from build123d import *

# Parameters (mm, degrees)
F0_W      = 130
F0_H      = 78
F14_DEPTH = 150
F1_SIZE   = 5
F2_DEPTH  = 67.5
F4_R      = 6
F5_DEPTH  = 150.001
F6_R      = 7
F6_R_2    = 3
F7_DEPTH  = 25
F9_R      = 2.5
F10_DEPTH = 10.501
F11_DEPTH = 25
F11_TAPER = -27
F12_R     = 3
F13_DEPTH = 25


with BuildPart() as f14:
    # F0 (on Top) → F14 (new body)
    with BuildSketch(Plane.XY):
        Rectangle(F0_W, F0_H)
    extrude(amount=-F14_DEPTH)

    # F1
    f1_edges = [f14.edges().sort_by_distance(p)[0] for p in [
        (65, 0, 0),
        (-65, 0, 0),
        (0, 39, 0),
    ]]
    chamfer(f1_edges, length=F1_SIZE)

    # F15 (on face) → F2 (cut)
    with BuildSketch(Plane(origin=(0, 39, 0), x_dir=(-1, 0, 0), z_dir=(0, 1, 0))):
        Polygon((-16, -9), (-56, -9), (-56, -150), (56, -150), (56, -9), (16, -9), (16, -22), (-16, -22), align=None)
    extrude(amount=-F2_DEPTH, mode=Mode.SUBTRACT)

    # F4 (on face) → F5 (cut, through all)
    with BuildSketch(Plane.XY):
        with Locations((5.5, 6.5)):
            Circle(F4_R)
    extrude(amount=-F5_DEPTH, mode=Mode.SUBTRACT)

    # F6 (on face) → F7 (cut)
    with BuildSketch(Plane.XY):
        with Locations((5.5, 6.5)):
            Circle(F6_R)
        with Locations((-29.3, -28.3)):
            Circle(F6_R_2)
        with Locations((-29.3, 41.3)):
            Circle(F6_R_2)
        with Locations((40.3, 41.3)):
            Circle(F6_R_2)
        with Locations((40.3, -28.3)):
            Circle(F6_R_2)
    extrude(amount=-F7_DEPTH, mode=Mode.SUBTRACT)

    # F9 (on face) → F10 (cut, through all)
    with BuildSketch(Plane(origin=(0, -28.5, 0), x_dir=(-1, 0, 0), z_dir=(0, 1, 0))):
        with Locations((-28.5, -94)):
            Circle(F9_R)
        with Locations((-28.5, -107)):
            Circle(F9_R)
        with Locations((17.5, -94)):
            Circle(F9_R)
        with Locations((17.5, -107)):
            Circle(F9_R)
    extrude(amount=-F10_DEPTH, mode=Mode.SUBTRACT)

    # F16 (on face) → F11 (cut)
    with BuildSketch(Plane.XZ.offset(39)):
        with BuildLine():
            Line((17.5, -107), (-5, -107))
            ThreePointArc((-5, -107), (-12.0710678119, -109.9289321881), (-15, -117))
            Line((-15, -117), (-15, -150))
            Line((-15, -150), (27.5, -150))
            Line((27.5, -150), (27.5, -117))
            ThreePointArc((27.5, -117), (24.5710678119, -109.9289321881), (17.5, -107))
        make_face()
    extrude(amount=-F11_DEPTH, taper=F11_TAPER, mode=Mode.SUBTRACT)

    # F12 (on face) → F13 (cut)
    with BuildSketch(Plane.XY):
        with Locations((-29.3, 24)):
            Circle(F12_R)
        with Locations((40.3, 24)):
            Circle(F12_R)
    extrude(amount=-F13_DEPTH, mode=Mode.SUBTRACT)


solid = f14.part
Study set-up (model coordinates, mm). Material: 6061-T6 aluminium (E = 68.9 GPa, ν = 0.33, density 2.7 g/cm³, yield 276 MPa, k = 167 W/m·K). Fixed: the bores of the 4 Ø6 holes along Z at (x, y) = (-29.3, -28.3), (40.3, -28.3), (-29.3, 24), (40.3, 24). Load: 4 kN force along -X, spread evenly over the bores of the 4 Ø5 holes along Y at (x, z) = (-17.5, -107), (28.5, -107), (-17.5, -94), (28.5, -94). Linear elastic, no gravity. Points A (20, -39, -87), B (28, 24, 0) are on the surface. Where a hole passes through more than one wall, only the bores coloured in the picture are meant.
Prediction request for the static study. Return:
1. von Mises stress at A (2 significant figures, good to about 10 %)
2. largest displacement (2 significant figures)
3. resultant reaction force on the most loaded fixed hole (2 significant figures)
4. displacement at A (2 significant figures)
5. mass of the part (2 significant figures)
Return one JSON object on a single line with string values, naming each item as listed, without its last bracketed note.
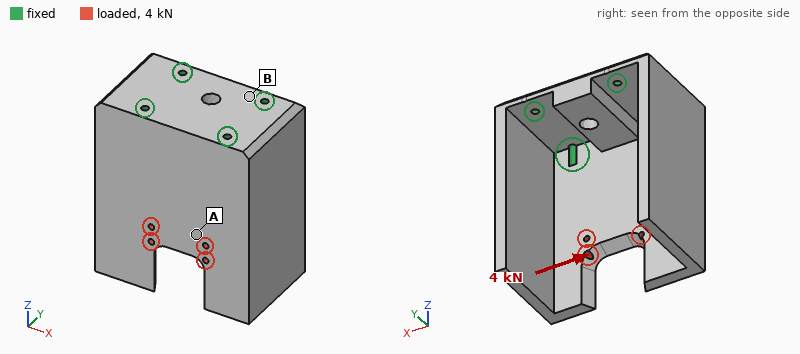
{"von Mises stress at A": "6.3 MPa", "largest displacement": "50 µm", "resultant reaction force on the most loaded fixed hole": "4.4 kN", "displacement at A": "20 µm", "mass of the part": "1.2 kg"}
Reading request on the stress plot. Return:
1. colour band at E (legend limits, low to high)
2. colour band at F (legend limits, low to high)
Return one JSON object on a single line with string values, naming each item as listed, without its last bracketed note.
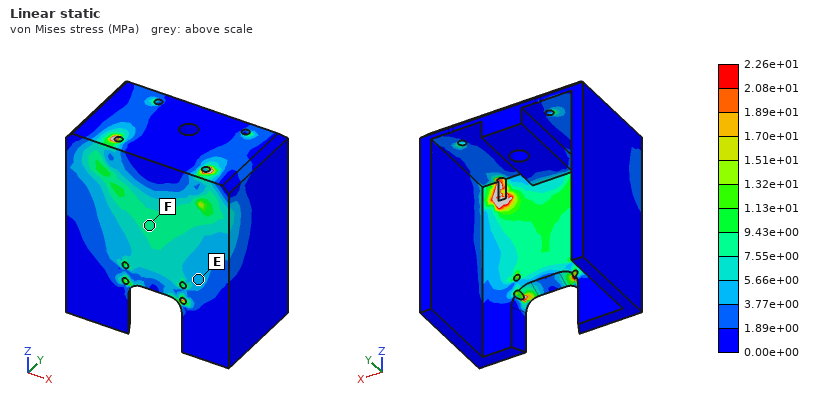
{"colour band at E": "3.77e+00 to 5.66e+00 MPa", "colour band at F": "7.55e+00 to 9.43e+00 MPa"}
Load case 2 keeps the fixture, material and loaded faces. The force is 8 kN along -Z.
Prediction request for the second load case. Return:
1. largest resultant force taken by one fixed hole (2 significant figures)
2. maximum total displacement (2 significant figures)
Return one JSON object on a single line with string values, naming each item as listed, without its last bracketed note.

{"largest resultant force taken by one fixed hole": "4.2 kN", "maximum total displacement": "27 µm"}
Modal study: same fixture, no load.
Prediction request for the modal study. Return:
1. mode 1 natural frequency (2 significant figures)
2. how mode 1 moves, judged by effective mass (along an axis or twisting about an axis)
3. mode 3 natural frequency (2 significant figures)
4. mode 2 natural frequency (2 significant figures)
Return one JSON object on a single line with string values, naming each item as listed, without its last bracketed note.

{"mode 1 natural frequency": "950 Hz", "how mode 1 moves, judged by effective mass": "along Y", "mode 3 natural frequency": "1200 Hz", "mode 2 natural frequency": "1100 Hz"}
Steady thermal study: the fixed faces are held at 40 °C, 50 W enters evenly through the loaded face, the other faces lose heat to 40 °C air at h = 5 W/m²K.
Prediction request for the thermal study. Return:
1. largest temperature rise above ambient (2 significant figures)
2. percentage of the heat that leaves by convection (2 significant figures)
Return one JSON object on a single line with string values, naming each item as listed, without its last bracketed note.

{"largest temperature rise above ambient": "18 K", "percentage of the heat that leaves by convection": "6.0 %"}
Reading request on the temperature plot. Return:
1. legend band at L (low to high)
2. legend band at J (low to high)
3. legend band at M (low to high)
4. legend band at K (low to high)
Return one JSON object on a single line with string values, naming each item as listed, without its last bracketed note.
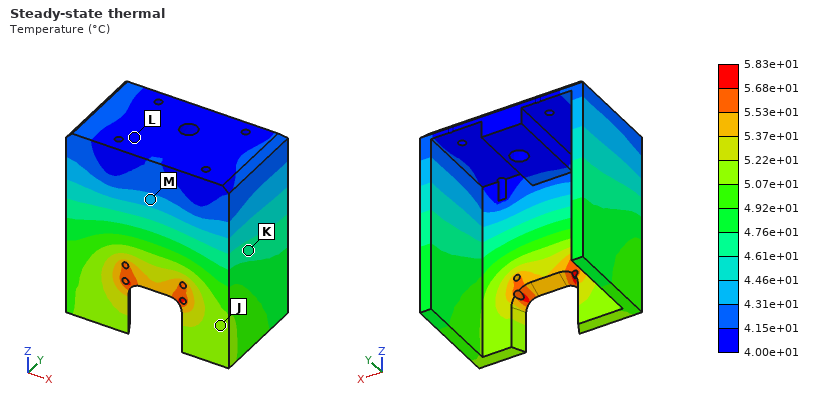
{"legend band at L": "4.00e+01 to 4.15e+01 °C", "legend band at J": "5.07e+01 to 5.22e+01 °C", "legend band at M": "4.31e+01 to 4.46e+01 °C", "legend band at K": "4.61e+01 to 4.76e+01 °C"}
